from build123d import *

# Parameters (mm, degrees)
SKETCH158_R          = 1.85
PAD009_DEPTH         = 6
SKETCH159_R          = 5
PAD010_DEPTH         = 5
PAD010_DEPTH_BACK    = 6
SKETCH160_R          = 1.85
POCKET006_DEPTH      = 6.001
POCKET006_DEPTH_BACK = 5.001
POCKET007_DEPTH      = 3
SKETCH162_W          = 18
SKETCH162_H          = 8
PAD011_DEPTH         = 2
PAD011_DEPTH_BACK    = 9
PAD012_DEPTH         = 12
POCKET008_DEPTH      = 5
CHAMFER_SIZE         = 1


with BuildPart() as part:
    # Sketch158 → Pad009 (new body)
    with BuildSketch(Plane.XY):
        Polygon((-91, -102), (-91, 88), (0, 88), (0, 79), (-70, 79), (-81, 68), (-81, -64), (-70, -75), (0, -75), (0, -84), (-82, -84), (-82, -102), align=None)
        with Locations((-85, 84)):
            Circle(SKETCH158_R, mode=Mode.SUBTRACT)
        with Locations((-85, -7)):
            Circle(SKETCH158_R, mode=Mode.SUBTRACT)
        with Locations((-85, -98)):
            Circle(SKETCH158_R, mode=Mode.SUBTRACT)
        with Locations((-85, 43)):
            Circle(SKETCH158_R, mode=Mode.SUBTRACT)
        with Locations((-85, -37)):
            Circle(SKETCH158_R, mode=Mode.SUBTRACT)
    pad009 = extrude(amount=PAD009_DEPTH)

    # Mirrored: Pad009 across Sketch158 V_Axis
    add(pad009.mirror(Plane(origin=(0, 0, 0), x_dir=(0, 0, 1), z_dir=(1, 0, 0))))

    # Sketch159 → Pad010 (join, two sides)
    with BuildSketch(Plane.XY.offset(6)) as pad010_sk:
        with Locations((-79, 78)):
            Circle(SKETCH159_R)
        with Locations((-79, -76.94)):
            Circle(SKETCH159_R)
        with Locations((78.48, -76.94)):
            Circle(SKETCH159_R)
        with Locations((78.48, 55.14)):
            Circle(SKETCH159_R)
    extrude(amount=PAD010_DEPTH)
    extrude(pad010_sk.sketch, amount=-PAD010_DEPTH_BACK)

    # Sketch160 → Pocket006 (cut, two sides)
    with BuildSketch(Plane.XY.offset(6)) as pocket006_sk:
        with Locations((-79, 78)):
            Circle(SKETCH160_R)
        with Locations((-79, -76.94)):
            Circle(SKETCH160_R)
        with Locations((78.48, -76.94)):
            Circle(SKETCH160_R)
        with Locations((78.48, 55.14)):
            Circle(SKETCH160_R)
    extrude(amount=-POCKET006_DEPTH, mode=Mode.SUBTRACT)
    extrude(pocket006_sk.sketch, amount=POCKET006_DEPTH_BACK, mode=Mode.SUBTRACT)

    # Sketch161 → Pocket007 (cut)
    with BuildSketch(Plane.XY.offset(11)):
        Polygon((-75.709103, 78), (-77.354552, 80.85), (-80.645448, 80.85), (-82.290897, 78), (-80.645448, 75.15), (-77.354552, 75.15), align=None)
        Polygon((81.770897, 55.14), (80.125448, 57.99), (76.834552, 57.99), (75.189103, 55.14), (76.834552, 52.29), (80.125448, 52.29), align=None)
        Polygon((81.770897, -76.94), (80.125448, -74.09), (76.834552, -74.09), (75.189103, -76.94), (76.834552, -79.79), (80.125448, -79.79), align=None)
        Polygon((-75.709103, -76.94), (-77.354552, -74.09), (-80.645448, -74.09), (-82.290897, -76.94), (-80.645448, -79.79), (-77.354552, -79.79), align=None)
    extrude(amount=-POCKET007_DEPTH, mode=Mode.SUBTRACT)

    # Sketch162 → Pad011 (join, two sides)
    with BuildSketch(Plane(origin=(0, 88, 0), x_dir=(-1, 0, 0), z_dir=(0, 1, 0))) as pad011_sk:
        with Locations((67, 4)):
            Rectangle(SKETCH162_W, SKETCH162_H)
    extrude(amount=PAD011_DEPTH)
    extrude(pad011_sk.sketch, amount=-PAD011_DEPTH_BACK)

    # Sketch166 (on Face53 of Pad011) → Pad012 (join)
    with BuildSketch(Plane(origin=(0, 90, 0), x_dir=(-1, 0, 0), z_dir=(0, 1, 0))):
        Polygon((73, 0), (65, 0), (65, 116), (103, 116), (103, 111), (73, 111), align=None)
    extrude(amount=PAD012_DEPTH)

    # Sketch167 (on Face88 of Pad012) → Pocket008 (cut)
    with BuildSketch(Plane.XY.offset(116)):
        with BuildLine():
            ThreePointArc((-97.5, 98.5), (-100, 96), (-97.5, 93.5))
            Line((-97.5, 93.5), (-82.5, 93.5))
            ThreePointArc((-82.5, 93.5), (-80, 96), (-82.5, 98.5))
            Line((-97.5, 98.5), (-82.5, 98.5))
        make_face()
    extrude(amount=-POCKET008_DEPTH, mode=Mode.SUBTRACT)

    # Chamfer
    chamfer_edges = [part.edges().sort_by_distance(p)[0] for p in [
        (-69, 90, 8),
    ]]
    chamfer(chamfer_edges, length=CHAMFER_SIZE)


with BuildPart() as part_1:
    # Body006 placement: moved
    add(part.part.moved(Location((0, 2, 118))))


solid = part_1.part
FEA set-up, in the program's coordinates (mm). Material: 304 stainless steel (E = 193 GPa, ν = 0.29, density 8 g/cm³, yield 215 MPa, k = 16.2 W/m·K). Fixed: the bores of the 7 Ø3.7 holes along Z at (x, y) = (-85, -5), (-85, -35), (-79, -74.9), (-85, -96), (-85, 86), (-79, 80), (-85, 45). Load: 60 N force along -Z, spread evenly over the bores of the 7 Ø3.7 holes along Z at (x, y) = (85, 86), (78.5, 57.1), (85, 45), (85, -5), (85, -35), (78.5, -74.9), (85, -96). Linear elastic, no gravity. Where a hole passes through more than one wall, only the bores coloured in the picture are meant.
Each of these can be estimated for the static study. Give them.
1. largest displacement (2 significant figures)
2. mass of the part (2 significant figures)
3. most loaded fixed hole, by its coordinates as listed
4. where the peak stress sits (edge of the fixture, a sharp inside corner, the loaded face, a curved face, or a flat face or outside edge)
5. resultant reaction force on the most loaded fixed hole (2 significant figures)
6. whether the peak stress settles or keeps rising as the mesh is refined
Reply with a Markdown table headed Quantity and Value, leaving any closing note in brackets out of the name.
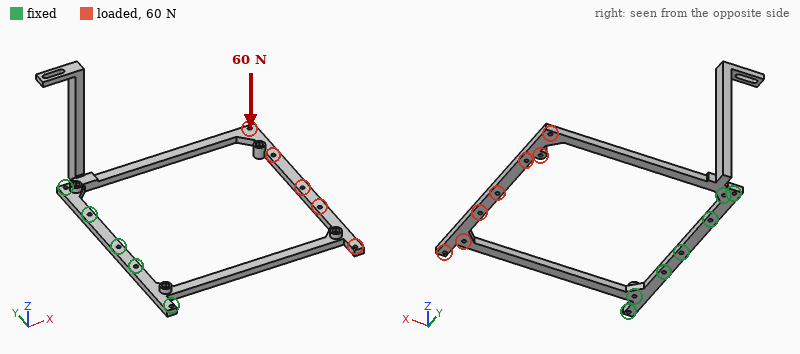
| Quantity | Value |
|---|---|
| largest displacement | 1.4 mm |
| mass of the part | 440 g |
| most loaded fixed hole, by its coordinates as listed | (-79, 80) |
| where the peak stress sits | a sharp inside corner |
| resultant reaction force on the most loaded fixed hole | 230 N |
| whether the peak stress settles or keeps rising as the mesh is refined | keeps rising |
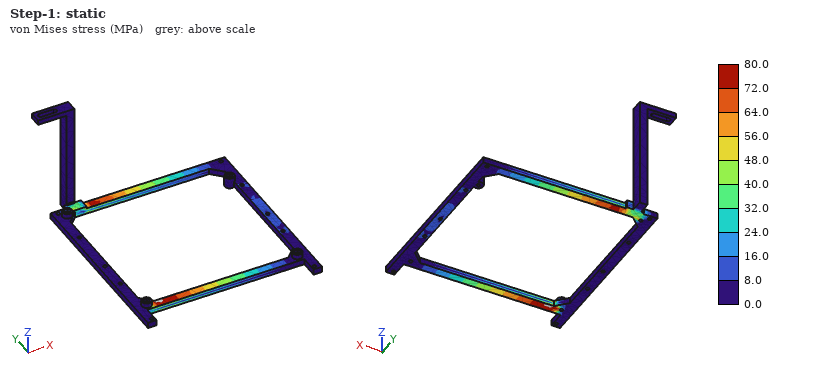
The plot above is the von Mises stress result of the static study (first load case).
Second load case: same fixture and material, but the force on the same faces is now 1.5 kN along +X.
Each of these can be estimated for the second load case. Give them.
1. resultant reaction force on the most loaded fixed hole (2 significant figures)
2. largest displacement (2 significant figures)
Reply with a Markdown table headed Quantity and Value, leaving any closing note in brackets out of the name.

| Quantity | Value |
|---|---|
| resultant reaction force on the most loaded fixed hole | 830 N |
| largest displacement | 0.27 mm |
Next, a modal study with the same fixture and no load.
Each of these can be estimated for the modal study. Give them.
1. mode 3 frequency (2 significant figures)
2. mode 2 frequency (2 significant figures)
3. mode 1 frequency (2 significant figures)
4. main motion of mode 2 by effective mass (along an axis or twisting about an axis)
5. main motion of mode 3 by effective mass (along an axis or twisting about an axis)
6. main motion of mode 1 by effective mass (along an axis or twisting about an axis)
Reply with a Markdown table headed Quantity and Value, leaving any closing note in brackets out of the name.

| Quantity | Value |
|---|---|
| mode 3 frequency | 260 Hz |
| mode 2 frequency | 220 Hz |
| mode 1 frequency | 97 Hz |
| main motion of mode 2 by effective mass | twisting about X |
| main motion of mode 3 by effective mass | along Y |
| main motion of mode 1 by effective mass | along Z |
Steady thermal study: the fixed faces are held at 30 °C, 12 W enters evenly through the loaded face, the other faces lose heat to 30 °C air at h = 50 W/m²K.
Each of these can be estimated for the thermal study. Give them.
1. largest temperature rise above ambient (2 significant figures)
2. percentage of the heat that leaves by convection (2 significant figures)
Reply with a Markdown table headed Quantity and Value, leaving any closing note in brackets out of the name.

| Quantity | Value |
|---|---|
| largest temperature rise above ambient | 47 K |
| percentage of the heat that leaves by convection | 100 % |
